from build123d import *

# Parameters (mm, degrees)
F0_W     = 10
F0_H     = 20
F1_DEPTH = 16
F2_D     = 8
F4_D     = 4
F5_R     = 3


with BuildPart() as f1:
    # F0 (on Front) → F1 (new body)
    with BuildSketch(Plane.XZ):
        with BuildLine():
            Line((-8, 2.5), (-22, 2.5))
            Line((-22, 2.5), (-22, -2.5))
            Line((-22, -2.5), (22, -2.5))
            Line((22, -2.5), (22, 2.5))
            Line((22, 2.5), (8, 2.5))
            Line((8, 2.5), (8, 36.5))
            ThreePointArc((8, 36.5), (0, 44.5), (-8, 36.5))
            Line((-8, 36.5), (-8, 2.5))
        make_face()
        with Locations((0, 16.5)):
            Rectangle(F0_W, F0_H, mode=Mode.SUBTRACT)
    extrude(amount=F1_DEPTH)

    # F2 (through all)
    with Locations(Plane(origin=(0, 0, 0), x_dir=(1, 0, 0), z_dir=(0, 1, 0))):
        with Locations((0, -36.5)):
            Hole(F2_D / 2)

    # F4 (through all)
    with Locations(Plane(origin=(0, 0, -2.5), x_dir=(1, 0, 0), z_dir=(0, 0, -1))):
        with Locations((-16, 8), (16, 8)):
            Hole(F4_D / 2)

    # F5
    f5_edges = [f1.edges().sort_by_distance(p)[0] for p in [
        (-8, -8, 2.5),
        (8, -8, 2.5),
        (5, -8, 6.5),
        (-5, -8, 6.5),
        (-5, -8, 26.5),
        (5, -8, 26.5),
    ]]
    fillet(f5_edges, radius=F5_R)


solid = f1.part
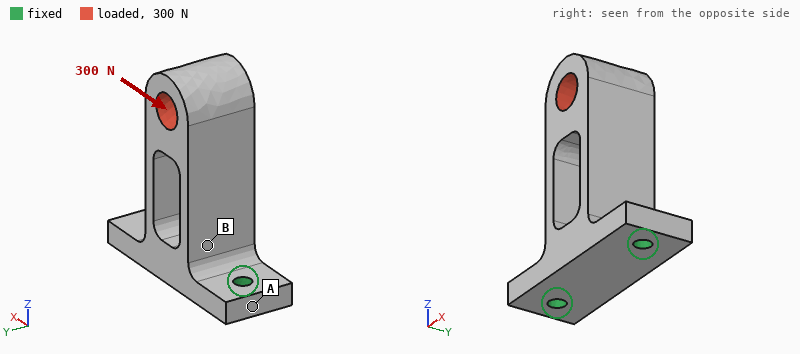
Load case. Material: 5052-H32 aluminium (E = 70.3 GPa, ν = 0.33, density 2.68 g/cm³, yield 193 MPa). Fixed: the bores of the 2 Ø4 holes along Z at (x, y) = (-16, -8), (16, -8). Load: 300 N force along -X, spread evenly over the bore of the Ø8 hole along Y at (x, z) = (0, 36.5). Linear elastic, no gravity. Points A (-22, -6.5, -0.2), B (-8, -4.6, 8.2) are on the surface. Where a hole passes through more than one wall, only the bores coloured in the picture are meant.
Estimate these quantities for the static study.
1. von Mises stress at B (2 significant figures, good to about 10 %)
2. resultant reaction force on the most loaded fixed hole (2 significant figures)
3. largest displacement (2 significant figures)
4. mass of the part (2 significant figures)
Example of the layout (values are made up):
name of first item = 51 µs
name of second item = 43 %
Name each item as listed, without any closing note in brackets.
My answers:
von Mises stress at B = 49 MPa
resultant reaction force on the most loaded fixed hole = 460 N
largest displacement = 73 µm
mass of the part = 26 g
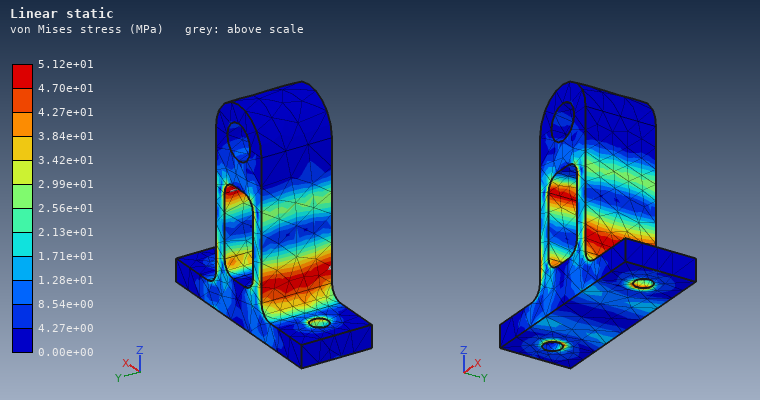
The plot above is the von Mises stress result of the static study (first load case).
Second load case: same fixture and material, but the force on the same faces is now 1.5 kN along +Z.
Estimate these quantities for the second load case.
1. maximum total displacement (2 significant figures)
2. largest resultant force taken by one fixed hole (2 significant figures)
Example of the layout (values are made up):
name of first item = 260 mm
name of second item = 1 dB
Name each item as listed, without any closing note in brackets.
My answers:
maximum total displacement = 15 µm
largest resultant force taken by one fixed hole = 810 N
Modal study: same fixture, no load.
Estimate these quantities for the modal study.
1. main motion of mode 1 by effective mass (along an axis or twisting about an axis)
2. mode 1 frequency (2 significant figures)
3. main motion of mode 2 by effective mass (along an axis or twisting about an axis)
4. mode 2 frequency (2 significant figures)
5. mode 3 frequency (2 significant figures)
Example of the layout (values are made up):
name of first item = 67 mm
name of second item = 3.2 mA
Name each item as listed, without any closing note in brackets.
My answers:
main motion of mode 1 by effective mass = along Y
mode 1 frequency = 2600 Hz
main motion of mode 2 by effective mass = along X
mode 2 frequency = 3400 Hz
mode 3 frequency = 9700 Hz
